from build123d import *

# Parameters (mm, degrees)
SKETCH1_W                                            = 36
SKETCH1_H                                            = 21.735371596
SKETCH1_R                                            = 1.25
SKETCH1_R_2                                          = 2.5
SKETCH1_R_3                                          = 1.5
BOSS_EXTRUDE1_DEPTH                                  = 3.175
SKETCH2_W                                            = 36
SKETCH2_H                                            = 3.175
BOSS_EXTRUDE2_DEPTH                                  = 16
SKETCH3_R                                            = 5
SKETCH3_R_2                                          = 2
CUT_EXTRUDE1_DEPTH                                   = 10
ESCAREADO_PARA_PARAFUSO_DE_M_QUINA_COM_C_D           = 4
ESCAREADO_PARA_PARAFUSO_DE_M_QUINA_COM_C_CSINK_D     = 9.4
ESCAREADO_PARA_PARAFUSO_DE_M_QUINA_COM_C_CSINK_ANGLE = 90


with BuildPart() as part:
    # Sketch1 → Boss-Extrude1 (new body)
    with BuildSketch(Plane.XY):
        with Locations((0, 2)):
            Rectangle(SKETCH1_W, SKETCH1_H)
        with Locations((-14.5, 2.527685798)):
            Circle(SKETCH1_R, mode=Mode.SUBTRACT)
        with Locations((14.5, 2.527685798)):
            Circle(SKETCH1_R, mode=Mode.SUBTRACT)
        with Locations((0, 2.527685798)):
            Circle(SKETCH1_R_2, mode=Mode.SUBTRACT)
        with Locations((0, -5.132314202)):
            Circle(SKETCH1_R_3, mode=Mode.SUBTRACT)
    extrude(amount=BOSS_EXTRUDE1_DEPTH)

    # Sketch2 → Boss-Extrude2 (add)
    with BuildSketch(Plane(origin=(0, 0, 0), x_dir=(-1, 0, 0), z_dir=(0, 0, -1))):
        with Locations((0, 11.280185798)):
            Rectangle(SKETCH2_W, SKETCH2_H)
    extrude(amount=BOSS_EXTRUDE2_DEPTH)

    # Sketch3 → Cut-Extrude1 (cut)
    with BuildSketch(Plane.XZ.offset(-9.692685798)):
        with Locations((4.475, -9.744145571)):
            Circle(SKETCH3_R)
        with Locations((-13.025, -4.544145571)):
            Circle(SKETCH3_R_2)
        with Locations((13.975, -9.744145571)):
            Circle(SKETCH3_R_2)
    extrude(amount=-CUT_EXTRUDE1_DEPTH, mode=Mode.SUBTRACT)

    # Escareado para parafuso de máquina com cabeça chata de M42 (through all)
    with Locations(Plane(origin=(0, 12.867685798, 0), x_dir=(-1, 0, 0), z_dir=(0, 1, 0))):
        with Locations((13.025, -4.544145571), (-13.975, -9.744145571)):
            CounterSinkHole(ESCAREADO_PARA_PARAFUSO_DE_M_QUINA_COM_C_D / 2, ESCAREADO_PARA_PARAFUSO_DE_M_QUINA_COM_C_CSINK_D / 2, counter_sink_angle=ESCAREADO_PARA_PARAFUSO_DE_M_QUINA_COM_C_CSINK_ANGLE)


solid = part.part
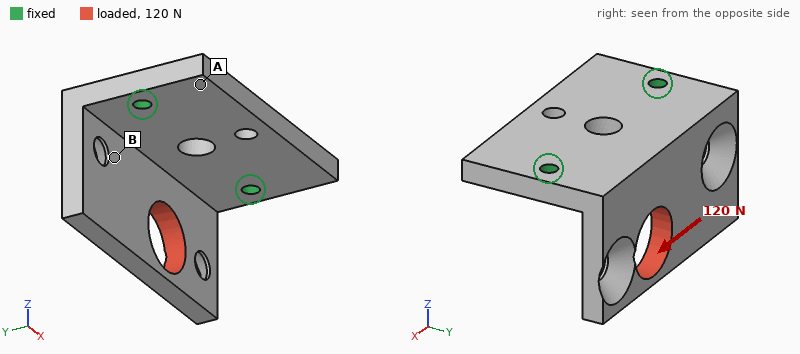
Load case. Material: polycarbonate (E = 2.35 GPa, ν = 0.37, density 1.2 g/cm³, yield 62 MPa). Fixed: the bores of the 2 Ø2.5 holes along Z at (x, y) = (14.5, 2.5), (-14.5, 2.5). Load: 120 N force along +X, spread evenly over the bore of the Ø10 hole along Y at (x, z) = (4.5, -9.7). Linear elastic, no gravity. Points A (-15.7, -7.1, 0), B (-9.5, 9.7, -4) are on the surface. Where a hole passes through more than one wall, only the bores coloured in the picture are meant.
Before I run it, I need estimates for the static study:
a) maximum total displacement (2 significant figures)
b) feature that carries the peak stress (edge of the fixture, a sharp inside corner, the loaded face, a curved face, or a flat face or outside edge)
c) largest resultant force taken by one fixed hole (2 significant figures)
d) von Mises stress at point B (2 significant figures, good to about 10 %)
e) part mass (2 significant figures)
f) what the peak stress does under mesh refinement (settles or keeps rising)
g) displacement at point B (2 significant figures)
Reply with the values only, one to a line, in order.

0.26 mm
edge of the fixture
85 N
5.8 MPa
4.5 g
keeps rising
0.093 mm
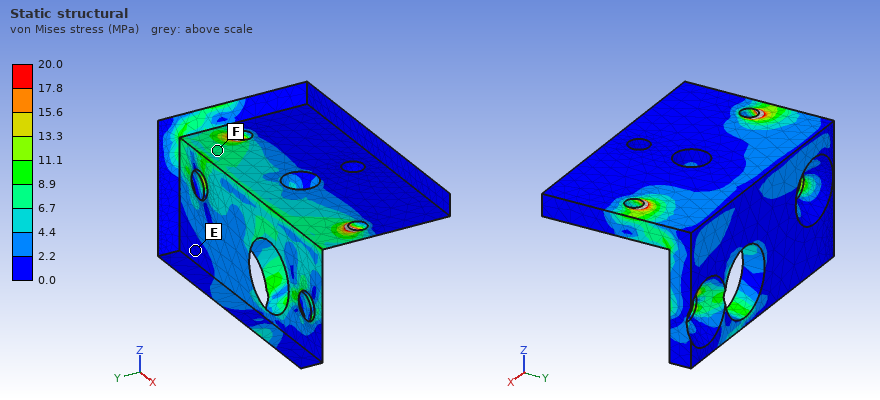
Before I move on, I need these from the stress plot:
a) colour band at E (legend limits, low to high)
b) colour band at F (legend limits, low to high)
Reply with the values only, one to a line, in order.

0.0 to 2.2 MPa
6.7 to 8.9 MPa
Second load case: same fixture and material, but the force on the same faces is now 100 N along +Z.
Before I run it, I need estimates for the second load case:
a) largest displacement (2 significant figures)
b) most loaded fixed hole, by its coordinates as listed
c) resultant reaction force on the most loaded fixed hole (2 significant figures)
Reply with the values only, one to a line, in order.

0.54 mm
(14.5, 2.5)
66 N
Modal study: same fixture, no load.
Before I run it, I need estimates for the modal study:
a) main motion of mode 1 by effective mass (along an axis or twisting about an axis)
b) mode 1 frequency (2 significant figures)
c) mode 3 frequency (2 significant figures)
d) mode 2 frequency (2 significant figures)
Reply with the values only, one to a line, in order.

along Y
1300 Hz
3400 Hz
2300 Hz
